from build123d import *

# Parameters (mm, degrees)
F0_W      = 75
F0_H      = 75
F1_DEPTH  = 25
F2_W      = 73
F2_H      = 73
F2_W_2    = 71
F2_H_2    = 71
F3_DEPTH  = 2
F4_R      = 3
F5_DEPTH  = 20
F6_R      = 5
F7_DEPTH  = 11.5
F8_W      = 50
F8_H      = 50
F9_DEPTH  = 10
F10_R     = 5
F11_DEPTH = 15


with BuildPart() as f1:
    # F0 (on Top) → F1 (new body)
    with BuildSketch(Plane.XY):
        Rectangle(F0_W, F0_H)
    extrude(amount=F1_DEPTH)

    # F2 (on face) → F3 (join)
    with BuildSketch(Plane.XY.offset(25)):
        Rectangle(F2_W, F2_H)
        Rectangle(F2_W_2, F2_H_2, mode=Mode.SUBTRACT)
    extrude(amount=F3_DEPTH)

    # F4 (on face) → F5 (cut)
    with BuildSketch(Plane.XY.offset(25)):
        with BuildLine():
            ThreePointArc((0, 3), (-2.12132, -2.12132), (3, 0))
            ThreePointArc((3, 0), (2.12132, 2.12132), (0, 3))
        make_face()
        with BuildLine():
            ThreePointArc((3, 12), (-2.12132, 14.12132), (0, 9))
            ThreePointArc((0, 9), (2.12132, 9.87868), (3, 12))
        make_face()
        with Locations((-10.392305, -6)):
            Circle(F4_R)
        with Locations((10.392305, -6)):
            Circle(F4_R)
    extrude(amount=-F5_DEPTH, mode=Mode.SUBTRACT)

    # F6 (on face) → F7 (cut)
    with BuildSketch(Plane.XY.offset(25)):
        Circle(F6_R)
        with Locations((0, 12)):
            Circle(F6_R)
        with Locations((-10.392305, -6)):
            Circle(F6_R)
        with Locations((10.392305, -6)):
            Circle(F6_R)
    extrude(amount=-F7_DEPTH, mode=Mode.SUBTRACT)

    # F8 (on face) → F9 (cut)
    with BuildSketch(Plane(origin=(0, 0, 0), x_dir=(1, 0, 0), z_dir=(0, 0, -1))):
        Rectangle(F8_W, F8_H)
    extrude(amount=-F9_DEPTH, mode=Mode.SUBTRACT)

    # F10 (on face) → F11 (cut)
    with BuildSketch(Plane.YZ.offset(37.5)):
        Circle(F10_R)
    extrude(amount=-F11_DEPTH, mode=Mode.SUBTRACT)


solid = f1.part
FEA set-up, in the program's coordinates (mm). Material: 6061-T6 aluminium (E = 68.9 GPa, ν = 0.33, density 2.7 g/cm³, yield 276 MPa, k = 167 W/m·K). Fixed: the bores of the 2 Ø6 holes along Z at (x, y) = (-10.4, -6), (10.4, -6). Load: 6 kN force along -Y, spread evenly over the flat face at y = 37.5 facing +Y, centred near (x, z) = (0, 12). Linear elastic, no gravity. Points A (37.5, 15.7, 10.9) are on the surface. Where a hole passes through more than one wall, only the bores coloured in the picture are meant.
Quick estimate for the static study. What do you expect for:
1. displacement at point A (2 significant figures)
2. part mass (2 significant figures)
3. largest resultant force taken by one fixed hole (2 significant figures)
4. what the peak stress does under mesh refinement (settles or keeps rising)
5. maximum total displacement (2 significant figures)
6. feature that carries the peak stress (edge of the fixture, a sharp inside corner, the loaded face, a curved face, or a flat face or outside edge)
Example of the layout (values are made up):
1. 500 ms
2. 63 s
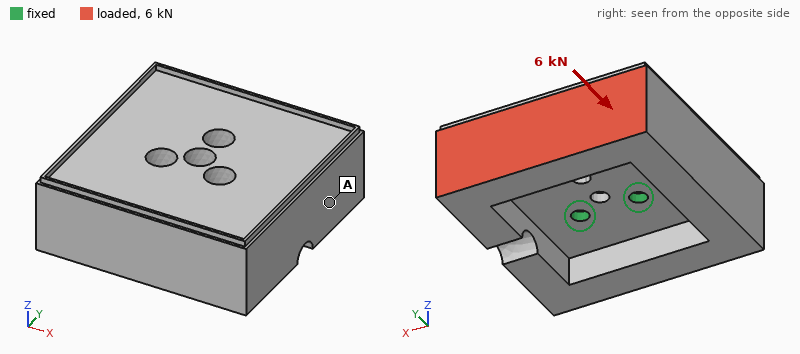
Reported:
1. 11 µm
2. 300 g
3. 3.0 kN
4. keeps rising
5. 19 µm
6. edge of the fixture
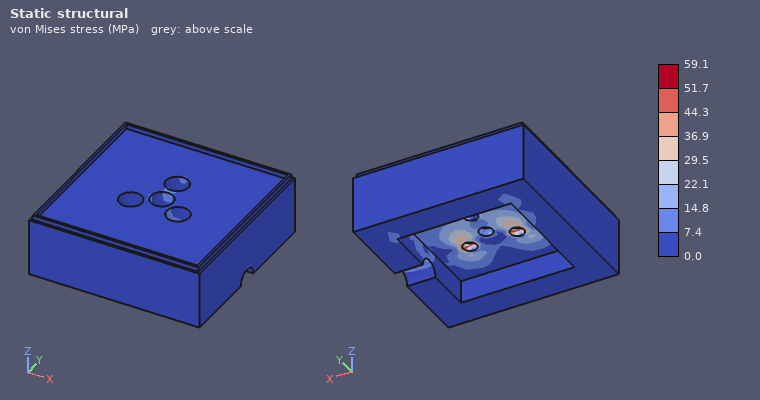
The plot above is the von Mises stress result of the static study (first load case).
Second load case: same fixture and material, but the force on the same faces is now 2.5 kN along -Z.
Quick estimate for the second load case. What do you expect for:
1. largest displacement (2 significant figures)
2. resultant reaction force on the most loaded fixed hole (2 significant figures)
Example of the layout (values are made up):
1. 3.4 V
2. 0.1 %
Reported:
1. 0.47 mm
2. 1.3 kN
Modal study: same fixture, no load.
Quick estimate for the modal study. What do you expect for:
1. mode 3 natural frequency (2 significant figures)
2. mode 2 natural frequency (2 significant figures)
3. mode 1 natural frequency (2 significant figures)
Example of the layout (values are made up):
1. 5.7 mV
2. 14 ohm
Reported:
1. 3300 Hz
2. 3200 Hz
3. 1200 Hz
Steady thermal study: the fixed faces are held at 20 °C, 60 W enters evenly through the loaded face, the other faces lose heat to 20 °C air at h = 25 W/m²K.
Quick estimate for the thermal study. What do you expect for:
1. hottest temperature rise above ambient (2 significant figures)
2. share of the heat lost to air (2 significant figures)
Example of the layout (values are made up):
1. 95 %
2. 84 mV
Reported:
1. 20 K
2. 9.8 %
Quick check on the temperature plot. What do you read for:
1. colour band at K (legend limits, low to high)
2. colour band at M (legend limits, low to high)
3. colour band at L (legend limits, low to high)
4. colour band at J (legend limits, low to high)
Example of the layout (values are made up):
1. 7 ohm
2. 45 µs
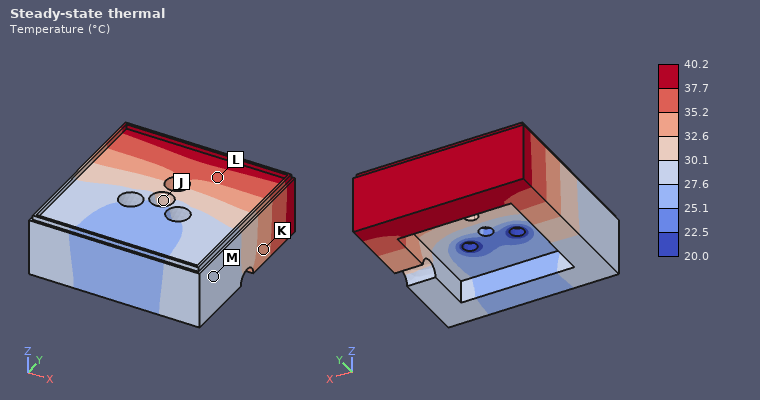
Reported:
1. 32.6 to 35.2 °C
2. 27.6 to 30.1 °C
3. 35.2 to 37.7 °C
4. 30.1 to 32.6 °C
